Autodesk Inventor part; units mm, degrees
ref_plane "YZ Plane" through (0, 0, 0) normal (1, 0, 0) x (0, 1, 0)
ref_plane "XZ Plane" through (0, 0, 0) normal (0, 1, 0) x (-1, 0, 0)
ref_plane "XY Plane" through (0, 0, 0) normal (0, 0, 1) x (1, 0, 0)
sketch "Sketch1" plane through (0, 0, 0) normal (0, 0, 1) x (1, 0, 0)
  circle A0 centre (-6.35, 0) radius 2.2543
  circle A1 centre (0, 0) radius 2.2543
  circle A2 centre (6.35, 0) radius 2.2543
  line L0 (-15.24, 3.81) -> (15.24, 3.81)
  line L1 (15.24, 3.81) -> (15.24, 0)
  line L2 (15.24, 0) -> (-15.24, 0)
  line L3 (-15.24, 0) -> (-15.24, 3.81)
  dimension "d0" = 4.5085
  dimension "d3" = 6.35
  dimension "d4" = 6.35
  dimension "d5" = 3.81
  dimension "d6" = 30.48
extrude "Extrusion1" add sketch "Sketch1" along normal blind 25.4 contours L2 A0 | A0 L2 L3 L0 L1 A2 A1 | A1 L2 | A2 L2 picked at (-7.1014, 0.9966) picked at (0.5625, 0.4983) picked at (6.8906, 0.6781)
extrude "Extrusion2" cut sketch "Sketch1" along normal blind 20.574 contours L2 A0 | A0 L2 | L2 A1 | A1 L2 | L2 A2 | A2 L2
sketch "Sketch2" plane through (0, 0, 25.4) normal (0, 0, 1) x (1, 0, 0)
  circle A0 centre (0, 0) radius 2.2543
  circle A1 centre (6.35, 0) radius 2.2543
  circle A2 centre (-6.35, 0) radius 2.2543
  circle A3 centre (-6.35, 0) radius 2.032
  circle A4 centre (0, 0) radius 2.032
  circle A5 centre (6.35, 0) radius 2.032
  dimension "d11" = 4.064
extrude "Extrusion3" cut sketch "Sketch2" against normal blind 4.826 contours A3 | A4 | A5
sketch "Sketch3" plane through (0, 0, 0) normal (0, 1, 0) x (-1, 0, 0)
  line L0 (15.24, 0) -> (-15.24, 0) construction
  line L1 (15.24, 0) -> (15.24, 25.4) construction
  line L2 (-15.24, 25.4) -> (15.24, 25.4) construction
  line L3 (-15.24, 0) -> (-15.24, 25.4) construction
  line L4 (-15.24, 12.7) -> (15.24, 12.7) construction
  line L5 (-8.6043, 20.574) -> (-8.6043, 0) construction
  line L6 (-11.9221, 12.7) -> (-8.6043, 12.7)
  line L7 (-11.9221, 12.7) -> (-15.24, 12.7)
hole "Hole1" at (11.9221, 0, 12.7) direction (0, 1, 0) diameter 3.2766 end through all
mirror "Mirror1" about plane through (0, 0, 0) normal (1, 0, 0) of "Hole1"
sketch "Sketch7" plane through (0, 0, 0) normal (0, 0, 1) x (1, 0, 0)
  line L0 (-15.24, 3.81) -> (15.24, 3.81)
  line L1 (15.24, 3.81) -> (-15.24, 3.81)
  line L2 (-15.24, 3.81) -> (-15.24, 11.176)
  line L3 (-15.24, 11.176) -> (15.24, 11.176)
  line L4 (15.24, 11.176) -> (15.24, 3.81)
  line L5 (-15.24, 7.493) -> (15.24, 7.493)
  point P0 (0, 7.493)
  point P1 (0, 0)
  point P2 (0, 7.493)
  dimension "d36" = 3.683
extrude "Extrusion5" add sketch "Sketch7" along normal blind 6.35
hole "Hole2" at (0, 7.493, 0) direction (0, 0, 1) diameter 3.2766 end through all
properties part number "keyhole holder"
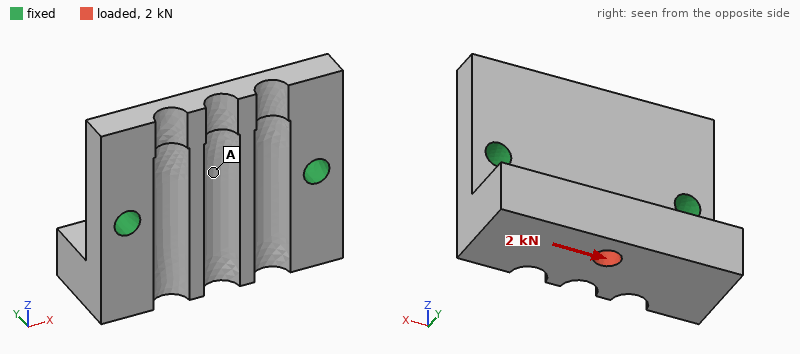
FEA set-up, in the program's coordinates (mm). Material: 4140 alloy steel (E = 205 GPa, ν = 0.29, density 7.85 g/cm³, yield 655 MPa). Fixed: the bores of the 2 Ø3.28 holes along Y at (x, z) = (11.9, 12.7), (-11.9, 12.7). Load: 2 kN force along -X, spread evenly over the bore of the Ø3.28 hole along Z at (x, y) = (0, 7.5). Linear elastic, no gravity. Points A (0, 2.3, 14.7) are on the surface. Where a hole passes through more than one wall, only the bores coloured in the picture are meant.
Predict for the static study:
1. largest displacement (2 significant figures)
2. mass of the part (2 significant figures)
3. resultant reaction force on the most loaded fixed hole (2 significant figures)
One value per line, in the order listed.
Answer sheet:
9.3 µm
29 g
1.3 kN
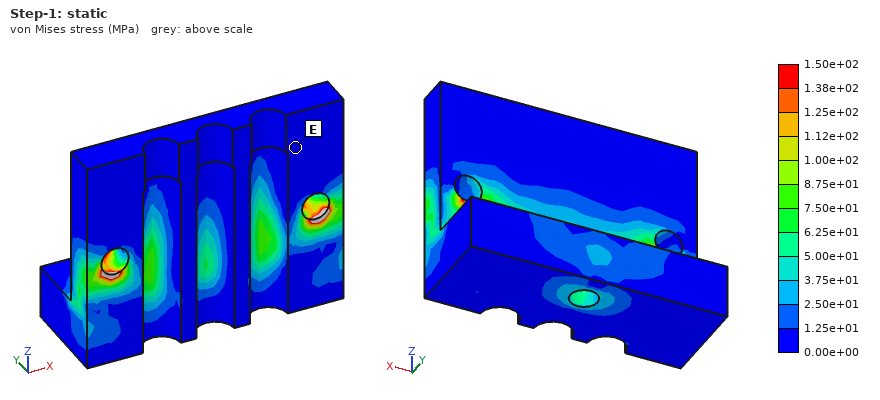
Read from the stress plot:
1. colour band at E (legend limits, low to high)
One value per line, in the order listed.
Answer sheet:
0.00e+00 to 1.25e+01 MPa
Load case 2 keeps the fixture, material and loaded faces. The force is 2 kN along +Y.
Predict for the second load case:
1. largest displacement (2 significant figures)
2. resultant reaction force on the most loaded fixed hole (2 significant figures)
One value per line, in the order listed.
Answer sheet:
62 µm
1.0 kN
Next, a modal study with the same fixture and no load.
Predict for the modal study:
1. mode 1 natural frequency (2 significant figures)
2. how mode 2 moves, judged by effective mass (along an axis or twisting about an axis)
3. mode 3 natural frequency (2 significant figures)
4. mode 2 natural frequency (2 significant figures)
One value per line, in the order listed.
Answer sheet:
8200 Hz
along Y
17 kHz
16 kHz
